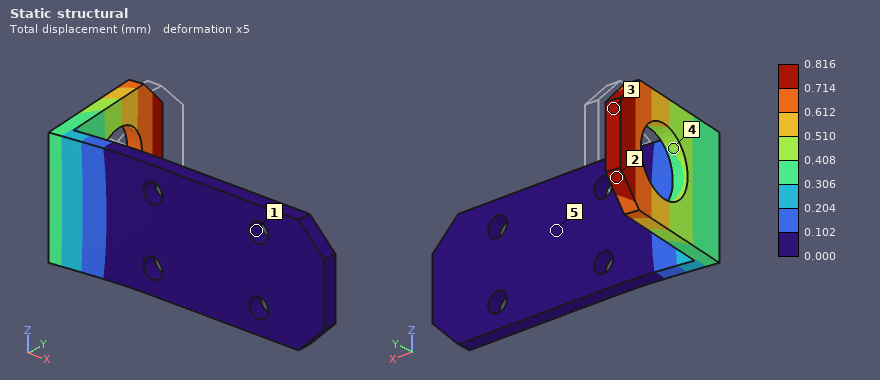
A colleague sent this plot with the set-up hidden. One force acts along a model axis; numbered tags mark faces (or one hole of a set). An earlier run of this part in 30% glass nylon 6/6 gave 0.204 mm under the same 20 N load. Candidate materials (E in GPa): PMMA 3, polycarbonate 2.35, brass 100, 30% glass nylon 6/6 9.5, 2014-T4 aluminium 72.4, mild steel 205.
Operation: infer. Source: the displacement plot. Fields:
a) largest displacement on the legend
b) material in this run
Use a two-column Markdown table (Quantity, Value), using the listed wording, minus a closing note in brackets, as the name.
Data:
| Quantity | Value |
|---|---|
| largest displacement on the legend | 0.816 mm |
| material in this run | polycarbonate |
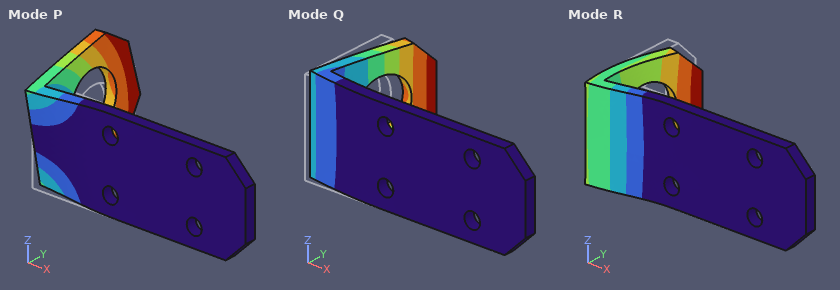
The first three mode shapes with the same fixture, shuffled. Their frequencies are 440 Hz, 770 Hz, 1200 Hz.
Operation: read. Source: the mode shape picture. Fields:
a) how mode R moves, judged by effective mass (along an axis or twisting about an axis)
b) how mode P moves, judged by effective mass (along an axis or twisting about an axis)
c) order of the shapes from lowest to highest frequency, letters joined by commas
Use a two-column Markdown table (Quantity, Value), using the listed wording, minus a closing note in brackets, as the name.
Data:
| Quantity | Value |
|---|---|
| how mode R moves, judged by effective mass | along Y |
| how mode P moves, judged by effective mass | along Z |
| order of the shapes from lowest to highest frequency, letters joined by commas | Q, P, R |
